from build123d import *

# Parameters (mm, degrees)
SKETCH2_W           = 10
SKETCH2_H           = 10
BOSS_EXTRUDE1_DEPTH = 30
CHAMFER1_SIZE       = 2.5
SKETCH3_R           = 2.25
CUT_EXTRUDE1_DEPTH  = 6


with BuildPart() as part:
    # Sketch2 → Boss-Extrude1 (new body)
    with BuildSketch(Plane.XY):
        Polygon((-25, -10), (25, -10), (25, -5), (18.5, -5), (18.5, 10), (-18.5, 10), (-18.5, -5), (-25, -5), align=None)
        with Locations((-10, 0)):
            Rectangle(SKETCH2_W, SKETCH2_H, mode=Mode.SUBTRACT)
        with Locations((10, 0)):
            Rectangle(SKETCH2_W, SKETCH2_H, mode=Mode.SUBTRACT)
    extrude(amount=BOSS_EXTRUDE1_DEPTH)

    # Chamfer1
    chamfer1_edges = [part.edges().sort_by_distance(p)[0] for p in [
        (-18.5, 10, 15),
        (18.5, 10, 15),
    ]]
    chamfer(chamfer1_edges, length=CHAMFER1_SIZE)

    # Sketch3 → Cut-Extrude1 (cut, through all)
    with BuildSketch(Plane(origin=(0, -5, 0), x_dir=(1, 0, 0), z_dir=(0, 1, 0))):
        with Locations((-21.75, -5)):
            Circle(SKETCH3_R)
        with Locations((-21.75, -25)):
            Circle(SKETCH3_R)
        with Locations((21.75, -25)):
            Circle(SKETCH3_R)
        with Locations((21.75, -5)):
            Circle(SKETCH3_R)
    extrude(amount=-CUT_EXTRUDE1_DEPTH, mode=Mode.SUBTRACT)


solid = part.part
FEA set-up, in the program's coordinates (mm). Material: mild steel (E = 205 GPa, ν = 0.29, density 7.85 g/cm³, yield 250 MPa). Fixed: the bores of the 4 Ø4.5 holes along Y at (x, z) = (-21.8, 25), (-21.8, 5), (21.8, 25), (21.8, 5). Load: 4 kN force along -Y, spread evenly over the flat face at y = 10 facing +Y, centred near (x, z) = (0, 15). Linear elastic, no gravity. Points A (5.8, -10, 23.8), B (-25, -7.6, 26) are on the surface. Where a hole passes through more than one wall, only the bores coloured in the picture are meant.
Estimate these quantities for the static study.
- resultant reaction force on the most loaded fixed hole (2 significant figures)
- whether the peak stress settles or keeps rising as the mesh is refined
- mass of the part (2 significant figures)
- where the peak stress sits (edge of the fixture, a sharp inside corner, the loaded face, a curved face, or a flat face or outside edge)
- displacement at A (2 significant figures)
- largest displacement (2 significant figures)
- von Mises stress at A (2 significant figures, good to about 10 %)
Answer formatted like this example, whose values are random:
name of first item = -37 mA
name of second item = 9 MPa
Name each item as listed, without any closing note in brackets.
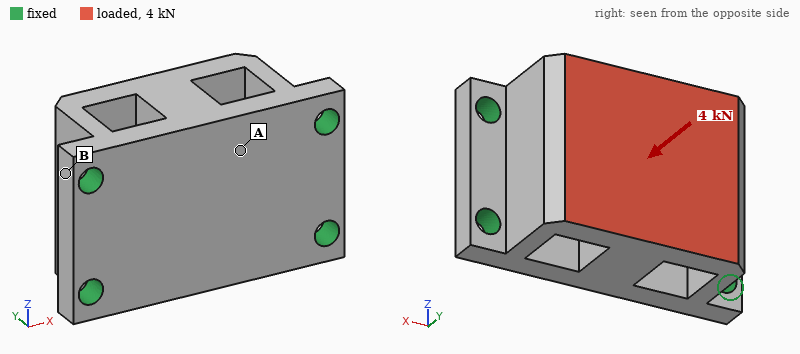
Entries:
resultant reaction force on the most loaded fixed hole = 1.1 kN
whether the peak stress settles or keeps rising as the mesh is refined = keeps rising
mass of the part = 140 g
where the peak stress sits = edge of the fixture
displacement at A = 5.9 µm
largest displacement = 6.9 µm
von Mises stress at A = 25 MPa
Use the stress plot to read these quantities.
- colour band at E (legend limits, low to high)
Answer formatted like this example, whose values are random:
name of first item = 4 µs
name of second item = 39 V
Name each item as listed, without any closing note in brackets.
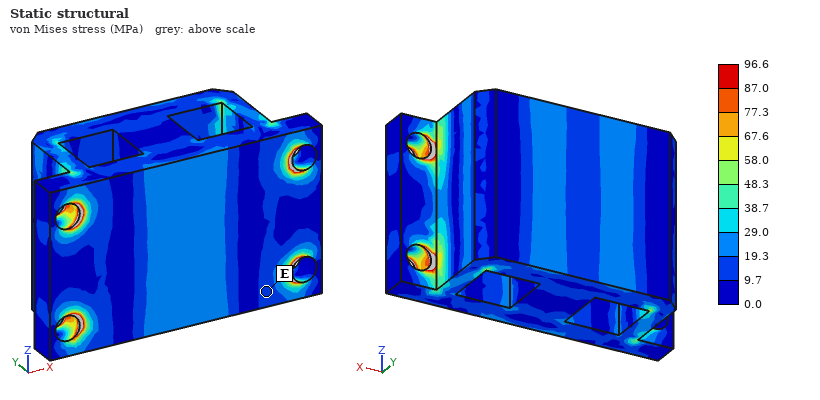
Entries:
colour band at E = 9.7 to 19.3 MPa
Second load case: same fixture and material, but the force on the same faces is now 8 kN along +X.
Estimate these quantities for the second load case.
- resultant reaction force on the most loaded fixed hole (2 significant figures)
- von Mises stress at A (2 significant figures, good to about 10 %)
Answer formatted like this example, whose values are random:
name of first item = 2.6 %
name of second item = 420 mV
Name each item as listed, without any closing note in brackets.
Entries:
resultant reaction force on the most loaded fixed hole = 2.8 kN
von Mises stress at A = 43 MPa
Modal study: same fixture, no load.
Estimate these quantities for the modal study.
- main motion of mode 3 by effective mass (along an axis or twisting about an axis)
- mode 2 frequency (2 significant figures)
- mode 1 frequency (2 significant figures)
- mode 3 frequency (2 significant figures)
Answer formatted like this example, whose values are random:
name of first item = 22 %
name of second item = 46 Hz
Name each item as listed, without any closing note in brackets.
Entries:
main motion of mode 3 by effective mass = along X
mode 2 frequency = 13 kHz
mode 1 frequency = 13 kHz
mode 3 frequency = 15 kHz
